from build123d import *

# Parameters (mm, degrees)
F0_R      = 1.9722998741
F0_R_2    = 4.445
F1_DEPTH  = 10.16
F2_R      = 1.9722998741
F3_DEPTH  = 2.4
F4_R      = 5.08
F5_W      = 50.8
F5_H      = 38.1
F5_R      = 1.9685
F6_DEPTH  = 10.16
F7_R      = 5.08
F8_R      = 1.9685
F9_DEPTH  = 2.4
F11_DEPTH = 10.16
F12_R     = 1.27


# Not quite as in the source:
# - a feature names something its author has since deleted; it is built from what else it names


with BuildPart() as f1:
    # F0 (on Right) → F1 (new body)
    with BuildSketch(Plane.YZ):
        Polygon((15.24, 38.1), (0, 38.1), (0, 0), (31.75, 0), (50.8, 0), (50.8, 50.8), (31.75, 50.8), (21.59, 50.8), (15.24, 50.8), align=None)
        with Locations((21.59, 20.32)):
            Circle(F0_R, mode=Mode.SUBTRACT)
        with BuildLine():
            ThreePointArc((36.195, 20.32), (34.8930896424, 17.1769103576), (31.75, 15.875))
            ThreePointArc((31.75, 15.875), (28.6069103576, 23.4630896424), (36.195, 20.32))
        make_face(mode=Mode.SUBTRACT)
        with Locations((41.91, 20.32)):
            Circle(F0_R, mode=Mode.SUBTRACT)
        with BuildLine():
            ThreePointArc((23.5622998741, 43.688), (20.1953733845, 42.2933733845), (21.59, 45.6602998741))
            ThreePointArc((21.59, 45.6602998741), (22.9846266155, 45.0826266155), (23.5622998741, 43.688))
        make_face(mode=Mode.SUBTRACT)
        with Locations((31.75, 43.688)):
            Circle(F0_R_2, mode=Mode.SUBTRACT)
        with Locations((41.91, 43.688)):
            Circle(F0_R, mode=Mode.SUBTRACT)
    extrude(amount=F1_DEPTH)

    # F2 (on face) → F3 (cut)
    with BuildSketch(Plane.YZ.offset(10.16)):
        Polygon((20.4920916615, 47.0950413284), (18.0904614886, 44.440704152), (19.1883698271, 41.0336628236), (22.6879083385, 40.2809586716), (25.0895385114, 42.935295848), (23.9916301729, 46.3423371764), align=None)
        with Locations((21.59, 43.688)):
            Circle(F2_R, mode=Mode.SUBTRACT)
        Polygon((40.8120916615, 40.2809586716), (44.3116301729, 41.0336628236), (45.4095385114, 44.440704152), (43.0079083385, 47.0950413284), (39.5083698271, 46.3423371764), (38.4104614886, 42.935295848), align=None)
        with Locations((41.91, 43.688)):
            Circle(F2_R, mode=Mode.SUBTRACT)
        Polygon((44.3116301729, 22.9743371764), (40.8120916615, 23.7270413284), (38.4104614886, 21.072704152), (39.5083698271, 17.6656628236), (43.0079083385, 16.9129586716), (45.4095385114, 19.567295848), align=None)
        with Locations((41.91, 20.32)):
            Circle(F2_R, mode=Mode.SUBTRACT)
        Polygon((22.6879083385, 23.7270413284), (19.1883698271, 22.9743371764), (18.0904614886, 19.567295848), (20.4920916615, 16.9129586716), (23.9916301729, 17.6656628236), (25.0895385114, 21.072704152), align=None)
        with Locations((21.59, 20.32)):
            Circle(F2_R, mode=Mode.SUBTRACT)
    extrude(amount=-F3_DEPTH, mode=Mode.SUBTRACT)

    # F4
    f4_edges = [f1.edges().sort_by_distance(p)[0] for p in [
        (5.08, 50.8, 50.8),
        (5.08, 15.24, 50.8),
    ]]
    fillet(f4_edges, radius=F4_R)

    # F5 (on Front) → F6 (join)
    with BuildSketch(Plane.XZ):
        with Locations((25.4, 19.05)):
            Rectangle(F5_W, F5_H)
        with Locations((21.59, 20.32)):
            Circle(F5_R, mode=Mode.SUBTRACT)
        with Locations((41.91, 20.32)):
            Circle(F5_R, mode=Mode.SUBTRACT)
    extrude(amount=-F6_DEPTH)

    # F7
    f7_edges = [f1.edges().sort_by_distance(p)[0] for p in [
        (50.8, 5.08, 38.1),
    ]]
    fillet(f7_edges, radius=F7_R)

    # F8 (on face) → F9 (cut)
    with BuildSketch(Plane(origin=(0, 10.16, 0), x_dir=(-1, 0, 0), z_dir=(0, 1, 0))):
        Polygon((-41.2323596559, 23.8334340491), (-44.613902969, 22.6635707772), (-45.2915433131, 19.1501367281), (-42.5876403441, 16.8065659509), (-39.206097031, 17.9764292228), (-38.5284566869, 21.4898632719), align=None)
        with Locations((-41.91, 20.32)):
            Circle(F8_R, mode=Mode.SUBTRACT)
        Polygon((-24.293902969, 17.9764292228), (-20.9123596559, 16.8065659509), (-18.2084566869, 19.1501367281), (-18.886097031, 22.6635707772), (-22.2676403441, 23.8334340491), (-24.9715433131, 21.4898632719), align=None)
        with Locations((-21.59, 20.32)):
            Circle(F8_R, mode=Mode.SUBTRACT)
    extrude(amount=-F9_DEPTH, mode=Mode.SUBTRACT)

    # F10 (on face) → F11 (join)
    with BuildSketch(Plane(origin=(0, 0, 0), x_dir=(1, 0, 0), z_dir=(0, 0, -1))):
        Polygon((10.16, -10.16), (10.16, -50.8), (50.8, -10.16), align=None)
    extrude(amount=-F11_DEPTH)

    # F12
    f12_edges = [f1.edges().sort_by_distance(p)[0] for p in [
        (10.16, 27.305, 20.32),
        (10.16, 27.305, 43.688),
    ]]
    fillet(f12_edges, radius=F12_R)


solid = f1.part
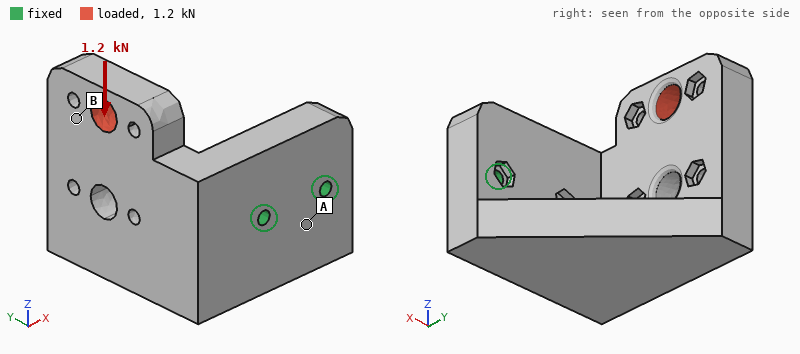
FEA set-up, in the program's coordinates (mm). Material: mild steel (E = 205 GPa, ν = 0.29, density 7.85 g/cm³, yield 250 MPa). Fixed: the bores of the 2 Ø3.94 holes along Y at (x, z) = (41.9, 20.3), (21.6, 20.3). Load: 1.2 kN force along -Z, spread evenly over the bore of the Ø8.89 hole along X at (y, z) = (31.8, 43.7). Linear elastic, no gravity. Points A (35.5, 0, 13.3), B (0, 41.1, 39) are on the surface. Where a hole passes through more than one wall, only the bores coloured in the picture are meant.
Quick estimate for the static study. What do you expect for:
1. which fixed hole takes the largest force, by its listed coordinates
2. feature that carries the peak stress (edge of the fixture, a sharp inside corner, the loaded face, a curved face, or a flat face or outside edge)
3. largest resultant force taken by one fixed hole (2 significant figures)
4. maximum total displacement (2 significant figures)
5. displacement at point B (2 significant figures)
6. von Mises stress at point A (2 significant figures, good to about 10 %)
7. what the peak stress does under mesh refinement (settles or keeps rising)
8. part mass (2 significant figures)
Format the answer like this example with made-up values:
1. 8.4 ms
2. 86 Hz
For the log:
1. (21.6, 20.3)
2. edge of the fixture
3. 2.0 kN
4. 41 µm
5. 32 µm
6. 26 MPa
7. keeps rising
8. 360 g
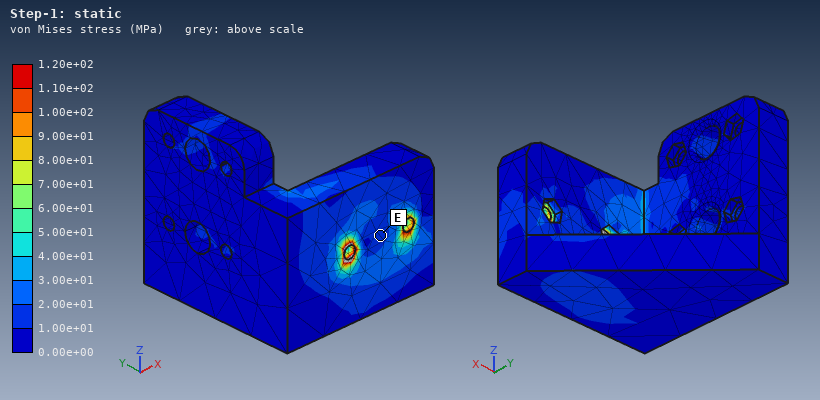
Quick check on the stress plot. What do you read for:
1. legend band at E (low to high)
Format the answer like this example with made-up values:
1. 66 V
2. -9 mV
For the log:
1. 1.00e+01 to 2.00e+01 MPa
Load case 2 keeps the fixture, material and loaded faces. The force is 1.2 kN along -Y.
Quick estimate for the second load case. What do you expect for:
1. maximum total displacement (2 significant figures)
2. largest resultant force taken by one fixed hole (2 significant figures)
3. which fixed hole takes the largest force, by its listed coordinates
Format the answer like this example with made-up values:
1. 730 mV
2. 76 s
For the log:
1. 38 µm
2. 1.8 kN
3. (21.6, 20.3)
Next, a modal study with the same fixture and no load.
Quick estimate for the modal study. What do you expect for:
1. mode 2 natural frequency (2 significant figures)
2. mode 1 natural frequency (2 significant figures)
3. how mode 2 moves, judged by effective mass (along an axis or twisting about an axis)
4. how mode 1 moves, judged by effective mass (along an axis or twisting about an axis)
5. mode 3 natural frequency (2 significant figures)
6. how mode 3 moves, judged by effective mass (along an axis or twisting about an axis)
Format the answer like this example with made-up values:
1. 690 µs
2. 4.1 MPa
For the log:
1. 3200 Hz
2. 2300 Hz
3. along X
4. along Z
5. 6300 Hz
6. along Y
